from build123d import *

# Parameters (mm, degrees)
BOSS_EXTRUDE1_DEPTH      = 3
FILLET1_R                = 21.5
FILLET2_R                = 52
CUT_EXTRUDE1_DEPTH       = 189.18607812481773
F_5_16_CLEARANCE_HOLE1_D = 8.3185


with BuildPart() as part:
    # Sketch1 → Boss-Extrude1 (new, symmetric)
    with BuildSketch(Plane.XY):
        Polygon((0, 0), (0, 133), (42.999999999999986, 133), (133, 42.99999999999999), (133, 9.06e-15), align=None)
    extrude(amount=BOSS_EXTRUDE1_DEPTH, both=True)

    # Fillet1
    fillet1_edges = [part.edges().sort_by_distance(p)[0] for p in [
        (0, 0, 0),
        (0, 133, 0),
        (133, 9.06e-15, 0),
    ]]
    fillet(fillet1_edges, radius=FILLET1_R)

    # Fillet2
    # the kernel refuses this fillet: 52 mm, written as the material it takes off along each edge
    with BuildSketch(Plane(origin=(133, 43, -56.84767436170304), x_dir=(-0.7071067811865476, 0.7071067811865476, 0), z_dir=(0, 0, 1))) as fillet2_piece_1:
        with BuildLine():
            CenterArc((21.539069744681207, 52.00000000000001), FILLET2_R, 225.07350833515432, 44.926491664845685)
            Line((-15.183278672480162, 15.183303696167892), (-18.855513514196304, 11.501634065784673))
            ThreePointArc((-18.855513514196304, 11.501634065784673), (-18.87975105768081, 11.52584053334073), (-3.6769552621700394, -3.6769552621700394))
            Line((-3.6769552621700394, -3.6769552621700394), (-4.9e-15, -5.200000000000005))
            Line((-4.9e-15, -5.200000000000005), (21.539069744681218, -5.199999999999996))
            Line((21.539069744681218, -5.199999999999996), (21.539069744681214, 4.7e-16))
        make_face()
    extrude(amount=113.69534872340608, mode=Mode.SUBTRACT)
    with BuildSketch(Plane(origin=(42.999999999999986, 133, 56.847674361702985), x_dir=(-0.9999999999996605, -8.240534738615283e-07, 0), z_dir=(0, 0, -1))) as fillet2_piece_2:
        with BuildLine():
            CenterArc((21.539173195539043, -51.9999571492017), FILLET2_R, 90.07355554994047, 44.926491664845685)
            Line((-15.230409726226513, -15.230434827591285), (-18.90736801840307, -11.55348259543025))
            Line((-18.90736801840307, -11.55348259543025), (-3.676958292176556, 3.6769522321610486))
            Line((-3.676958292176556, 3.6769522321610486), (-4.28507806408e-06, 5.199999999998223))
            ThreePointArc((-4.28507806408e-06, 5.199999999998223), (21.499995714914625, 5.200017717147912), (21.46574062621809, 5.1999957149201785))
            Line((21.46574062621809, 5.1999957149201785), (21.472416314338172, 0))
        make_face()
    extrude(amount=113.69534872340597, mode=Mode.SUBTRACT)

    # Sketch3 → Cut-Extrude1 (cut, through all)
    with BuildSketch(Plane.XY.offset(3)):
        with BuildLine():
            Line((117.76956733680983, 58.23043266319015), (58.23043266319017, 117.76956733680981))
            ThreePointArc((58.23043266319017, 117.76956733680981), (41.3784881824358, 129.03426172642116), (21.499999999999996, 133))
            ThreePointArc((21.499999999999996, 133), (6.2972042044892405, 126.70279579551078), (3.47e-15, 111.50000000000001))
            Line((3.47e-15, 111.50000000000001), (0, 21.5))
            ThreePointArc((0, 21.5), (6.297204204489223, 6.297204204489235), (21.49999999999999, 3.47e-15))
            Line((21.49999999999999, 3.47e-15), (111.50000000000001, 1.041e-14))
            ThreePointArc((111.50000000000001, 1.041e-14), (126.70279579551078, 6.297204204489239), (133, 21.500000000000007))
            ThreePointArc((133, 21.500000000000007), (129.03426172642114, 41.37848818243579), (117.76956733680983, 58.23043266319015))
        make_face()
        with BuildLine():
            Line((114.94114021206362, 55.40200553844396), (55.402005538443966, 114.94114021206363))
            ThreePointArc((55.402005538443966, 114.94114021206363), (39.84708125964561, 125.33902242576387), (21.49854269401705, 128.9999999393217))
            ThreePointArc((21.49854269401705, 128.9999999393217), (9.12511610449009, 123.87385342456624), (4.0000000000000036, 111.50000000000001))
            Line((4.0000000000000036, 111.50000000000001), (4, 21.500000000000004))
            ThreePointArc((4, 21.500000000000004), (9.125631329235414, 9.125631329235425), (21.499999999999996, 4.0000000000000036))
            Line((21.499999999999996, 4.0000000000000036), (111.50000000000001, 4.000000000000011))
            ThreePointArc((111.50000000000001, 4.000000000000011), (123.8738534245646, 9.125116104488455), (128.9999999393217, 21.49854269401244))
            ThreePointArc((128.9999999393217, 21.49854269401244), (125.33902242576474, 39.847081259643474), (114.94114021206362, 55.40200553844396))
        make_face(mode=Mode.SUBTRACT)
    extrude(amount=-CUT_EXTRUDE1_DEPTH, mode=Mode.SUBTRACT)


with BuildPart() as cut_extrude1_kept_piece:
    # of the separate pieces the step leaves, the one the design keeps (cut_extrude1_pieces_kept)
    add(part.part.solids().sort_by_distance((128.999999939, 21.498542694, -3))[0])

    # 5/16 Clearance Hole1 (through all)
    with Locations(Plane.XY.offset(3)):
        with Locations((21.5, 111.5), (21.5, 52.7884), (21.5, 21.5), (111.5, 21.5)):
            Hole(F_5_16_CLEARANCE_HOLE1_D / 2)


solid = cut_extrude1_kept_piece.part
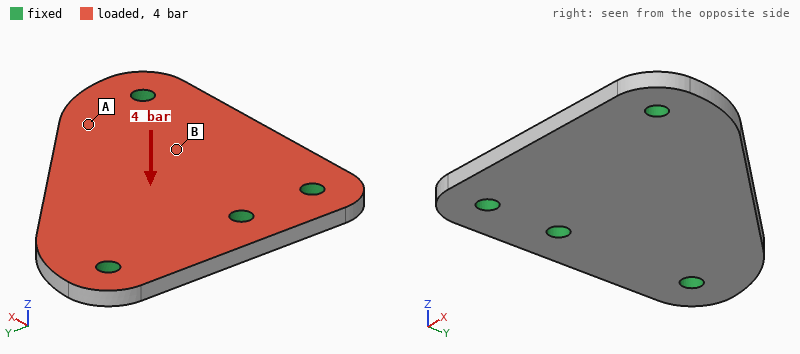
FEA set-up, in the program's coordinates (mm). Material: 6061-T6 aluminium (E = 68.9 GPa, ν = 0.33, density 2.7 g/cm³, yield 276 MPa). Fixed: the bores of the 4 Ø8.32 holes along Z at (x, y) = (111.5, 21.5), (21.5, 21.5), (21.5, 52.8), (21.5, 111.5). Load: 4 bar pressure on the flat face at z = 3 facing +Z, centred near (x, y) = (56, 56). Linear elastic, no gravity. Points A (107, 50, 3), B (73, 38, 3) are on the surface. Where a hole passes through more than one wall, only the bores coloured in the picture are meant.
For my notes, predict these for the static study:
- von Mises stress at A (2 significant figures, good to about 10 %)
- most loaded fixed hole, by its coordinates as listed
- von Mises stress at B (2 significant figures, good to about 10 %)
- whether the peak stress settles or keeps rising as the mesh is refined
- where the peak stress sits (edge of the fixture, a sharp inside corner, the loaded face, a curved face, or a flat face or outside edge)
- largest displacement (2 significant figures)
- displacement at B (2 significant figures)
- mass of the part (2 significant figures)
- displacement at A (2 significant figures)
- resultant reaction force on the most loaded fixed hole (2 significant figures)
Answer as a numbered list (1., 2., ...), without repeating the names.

1. 10 MPa
2. (111.5, 21.5)
3. 28 MPa
4. keeps rising
5. edge of the fixture
6. 0.23 mm
7. 0.084 mm
8. 180 g
9. 0.091 mm
10. 1.5 kN
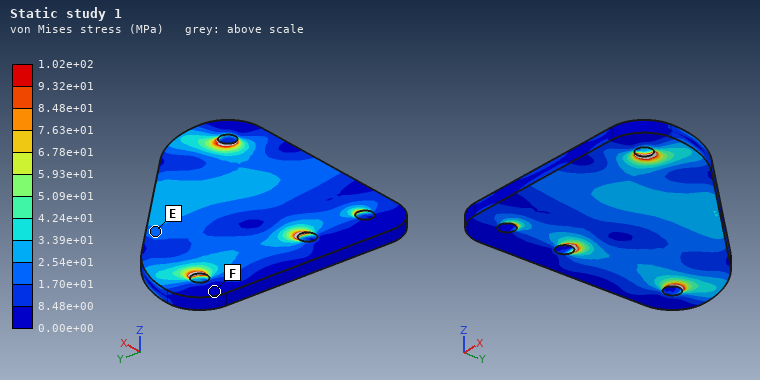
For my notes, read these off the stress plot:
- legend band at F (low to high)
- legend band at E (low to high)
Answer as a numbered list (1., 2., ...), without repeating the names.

1. 0.00e+00 to 8.48e+00 MPa
2. 1.70e+01 to 2.54e+01 MPa
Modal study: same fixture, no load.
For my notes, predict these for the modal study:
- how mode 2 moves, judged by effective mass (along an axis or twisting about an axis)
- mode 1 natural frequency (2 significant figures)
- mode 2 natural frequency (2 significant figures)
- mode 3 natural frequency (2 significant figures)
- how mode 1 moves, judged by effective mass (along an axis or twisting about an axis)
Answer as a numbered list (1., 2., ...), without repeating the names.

1. along Z
2. 2200 Hz
3. 4100 Hz
4. 5200 Hz
5. along Z
